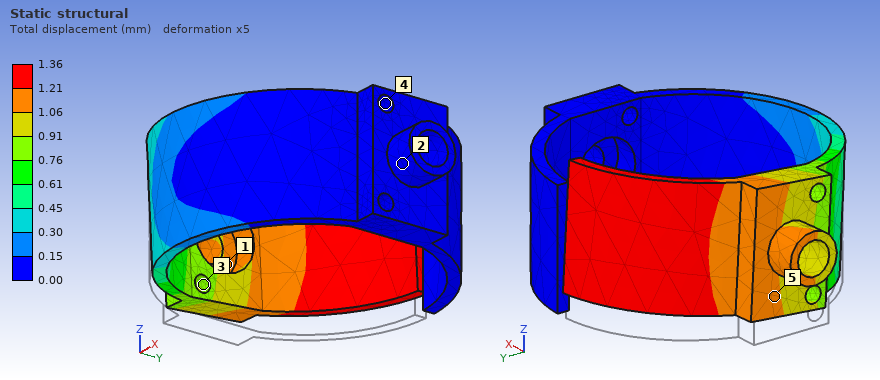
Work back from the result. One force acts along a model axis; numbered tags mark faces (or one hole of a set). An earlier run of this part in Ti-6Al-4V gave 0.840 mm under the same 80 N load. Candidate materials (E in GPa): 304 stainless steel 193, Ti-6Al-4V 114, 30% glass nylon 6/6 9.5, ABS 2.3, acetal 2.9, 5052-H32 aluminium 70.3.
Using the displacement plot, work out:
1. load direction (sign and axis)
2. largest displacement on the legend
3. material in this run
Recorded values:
+Z
1.36 mm
5052-H32 aluminium
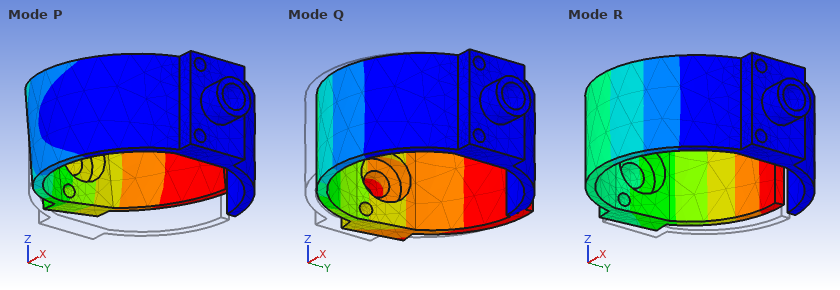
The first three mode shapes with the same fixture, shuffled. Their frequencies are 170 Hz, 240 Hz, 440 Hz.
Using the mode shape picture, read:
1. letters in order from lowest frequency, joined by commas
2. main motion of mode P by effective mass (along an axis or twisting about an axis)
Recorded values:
Q, P, R
along Z
